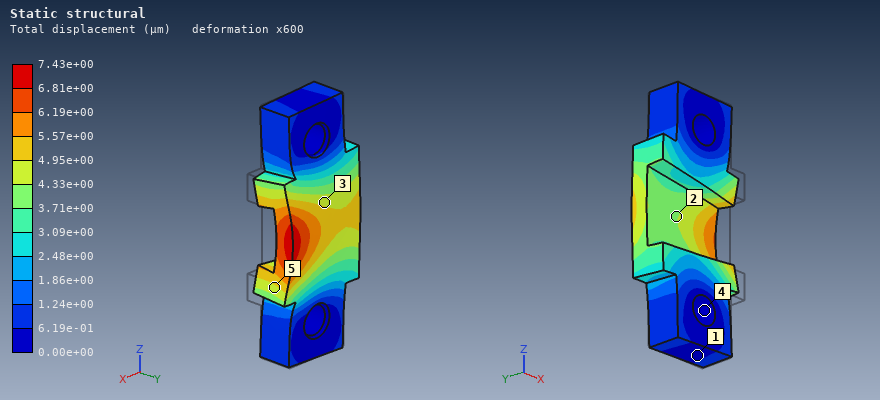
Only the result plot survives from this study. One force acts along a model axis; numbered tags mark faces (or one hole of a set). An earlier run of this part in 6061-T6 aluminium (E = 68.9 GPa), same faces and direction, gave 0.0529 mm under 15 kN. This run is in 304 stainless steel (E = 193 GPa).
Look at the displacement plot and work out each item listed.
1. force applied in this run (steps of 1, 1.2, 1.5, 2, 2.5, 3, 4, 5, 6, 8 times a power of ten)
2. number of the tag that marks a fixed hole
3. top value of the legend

6 kN
4
7.43e+00 µm
